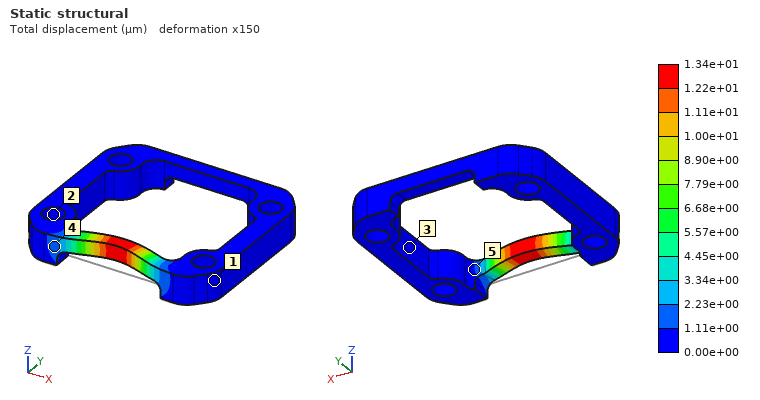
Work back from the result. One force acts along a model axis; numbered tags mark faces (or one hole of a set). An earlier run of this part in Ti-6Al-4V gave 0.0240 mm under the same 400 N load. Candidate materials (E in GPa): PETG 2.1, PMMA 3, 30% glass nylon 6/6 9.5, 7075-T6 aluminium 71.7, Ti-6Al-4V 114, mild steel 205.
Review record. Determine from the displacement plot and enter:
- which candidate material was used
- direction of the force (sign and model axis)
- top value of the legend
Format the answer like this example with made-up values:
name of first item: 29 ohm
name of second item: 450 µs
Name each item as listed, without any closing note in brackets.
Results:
which candidate material was used: mild steel
direction of the force: +Y
top value of the legend: 1.34e+01 µm
